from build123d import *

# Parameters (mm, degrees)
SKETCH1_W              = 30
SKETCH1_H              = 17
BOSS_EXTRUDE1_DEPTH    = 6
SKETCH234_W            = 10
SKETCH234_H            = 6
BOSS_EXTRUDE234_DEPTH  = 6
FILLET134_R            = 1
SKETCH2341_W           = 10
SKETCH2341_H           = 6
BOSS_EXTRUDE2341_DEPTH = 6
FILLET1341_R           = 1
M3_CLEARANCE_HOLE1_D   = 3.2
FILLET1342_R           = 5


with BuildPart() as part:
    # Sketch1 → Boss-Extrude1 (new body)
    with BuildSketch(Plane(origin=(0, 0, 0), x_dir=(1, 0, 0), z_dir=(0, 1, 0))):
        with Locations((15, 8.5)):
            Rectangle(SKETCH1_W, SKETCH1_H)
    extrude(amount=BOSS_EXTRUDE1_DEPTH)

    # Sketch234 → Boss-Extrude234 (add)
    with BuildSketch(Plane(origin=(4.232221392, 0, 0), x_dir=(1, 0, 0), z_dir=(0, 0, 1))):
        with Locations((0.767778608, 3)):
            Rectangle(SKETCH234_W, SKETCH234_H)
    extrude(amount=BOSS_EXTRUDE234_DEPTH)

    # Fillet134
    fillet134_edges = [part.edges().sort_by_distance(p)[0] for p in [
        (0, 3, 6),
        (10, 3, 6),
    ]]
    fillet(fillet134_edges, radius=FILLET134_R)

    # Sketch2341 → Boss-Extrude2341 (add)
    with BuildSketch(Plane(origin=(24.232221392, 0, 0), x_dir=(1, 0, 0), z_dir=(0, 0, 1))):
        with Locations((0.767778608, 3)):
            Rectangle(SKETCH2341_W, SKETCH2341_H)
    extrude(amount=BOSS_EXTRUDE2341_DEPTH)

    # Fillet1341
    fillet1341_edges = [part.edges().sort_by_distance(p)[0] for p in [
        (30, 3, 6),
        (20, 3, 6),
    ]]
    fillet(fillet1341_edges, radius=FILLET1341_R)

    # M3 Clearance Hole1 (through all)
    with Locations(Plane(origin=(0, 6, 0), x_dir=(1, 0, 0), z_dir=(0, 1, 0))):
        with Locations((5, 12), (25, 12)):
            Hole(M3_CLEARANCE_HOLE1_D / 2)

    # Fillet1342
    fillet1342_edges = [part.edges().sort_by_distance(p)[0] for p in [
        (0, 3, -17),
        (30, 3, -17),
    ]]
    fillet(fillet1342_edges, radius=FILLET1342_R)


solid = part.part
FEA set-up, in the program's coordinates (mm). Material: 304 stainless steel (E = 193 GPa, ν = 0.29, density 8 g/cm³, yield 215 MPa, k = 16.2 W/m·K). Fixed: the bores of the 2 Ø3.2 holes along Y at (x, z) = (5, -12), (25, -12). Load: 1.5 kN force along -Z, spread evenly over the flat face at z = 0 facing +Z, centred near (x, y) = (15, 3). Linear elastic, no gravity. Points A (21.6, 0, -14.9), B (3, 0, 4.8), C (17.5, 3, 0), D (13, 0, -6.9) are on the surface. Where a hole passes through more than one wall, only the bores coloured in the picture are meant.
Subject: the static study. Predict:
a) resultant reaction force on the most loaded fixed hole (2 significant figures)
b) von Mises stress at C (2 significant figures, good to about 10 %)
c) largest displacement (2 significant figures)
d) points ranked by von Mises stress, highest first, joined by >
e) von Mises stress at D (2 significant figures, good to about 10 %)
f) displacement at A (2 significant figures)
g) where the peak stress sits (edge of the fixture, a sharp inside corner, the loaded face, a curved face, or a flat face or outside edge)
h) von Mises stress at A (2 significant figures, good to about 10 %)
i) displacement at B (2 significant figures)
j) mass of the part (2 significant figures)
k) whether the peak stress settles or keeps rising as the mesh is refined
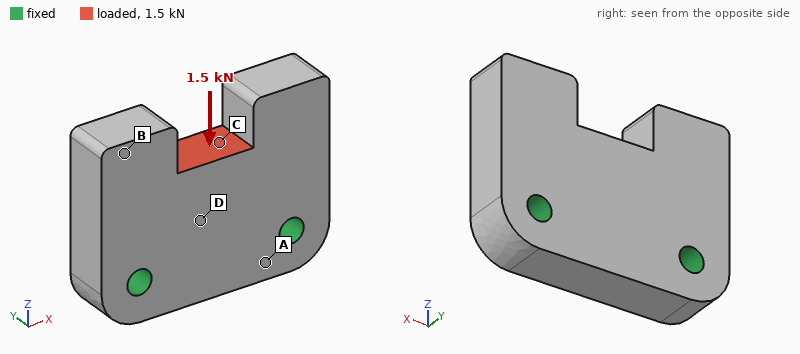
810 N
24 MPa
1.8 µm
C > D > A > B
14 MPa
0.41 µm
edge of the fixture
10 MPa
1.0 µm
29 g
keeps rising
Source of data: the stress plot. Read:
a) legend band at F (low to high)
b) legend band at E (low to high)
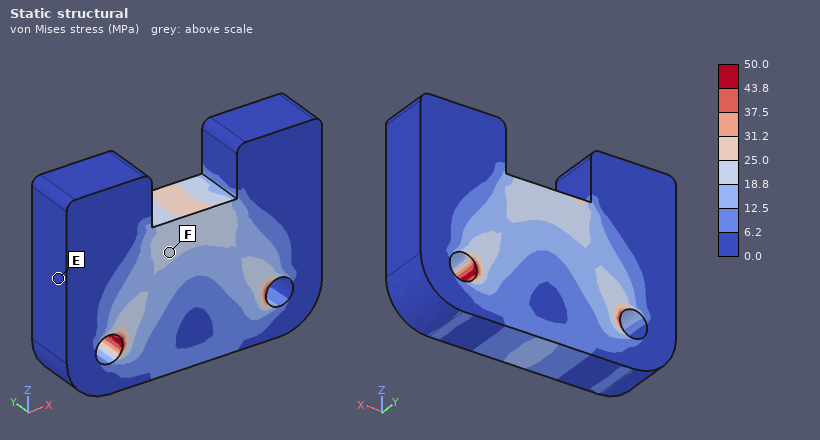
18.8 to 25.0 MPa
0.0 to 6.2 MPa
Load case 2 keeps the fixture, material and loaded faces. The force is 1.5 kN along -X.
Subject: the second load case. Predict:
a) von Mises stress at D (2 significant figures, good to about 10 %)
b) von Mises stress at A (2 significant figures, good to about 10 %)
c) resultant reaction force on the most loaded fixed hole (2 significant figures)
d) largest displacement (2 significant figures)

16 MPa
4.6 MPa
1.1 kN
2.5 µm
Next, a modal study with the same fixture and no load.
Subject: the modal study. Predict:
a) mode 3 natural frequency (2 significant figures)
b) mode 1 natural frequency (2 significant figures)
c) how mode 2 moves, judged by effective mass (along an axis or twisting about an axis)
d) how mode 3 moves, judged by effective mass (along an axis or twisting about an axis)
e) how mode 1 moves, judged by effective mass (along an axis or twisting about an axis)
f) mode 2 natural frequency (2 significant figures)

32 kHz
14 kHz
twisting about Z
along X
along Y
19 kHz
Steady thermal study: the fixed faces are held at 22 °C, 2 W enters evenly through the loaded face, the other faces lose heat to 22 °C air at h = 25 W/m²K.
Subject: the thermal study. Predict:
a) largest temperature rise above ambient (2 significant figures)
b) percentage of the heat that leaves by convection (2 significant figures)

15 K
9.3 %
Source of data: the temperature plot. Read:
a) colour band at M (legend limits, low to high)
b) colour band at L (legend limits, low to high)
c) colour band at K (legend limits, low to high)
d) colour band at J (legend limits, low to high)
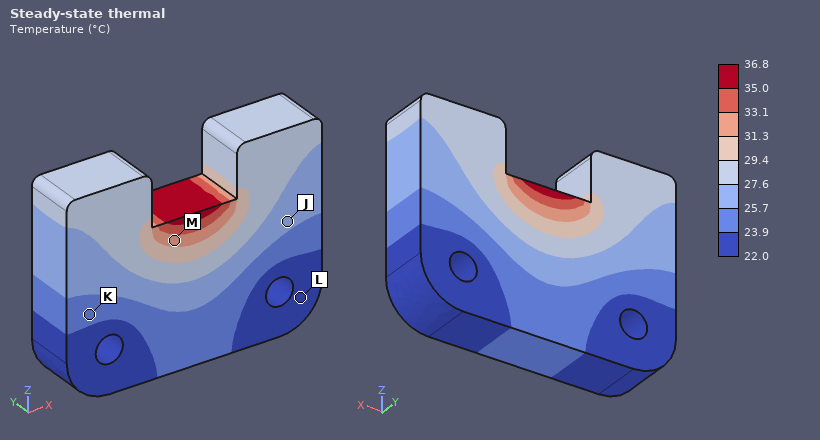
31.3 to 33.1 °C
22.0 to 23.9 °C
23.9 to 25.7 °C
25.7 to 27.6 °C
